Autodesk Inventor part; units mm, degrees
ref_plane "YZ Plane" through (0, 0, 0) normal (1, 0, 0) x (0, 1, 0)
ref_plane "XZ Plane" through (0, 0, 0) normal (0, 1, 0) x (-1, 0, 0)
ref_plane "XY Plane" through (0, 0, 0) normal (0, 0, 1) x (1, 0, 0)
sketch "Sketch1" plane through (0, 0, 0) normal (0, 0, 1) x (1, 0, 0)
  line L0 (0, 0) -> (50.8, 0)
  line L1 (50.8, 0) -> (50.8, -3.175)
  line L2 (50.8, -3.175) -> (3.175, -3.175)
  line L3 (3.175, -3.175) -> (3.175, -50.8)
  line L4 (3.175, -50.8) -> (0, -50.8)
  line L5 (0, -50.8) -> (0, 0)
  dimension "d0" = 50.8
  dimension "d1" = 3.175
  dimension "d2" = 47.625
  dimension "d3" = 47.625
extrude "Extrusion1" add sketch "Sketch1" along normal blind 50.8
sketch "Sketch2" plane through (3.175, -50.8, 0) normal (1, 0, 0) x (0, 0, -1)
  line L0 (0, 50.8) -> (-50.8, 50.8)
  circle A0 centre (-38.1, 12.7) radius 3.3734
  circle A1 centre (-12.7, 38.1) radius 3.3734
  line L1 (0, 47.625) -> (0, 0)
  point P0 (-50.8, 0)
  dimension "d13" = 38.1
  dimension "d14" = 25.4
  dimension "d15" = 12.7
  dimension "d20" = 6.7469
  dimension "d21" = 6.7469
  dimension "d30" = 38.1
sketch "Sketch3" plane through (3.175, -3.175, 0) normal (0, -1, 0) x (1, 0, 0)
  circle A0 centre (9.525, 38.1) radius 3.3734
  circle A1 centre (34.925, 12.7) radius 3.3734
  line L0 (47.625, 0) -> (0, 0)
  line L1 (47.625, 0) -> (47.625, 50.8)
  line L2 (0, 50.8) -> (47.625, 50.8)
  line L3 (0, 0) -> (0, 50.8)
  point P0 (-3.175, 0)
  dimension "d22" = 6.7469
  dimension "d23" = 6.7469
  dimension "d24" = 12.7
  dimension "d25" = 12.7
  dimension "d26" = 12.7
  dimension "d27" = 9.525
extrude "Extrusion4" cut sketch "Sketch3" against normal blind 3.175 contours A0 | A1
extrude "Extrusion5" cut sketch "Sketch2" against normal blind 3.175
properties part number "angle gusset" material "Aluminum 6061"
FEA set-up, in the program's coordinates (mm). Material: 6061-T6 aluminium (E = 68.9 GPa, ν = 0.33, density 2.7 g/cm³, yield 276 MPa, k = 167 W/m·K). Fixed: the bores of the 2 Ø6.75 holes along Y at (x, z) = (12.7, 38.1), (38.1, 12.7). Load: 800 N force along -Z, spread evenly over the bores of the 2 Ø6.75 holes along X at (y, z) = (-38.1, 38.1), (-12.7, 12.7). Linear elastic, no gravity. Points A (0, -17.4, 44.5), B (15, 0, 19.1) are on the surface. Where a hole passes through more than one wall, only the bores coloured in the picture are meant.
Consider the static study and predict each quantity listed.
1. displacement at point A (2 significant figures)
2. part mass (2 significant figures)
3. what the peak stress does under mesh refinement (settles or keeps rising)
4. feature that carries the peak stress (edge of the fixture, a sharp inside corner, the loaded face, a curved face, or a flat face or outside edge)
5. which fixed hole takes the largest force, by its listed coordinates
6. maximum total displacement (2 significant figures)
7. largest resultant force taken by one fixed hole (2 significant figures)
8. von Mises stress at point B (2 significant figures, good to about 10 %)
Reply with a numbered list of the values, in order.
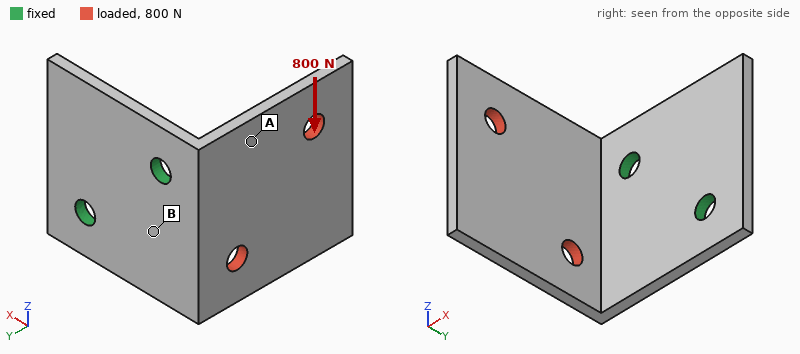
1. 0.19 mm
2. 42 g
3. keeps rising
4. edge of the fixture
5. (12.7, 38.1)
6. 0.80 mm
7. 860 N
8. 63 MPa
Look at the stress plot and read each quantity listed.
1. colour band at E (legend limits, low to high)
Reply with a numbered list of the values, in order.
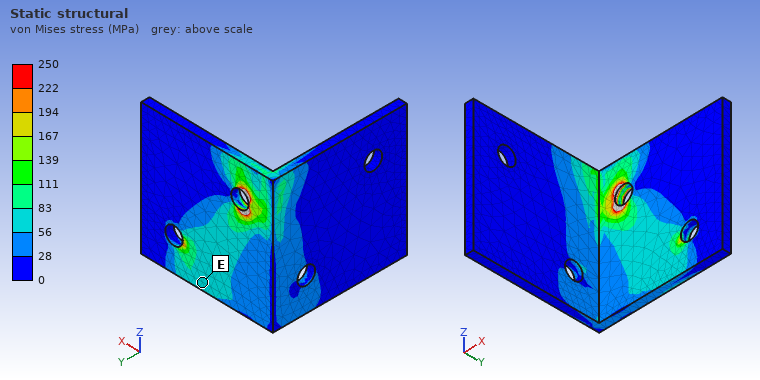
1. 56 to 83 MPa
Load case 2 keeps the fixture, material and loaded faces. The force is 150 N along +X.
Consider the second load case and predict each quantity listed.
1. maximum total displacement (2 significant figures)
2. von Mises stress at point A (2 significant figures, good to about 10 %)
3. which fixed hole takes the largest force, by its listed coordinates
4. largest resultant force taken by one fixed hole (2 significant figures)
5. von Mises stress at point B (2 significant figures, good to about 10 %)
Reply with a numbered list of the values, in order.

1. 0.45 mm
2. 23 MPa
3. (12.7, 38.1)
4. 94 N
5. 18 MPa
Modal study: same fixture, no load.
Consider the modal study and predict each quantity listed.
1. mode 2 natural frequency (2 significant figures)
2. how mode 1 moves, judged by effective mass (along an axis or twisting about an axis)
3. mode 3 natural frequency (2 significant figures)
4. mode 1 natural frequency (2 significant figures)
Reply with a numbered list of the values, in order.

1. 1300 Hz
2. along X
3. 2300 Hz
4. 770 Hz
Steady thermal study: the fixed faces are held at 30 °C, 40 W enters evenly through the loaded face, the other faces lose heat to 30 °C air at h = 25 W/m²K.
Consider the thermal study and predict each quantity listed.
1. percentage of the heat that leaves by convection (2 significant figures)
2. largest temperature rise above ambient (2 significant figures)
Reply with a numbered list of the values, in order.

1. 17 %
2. 62 K
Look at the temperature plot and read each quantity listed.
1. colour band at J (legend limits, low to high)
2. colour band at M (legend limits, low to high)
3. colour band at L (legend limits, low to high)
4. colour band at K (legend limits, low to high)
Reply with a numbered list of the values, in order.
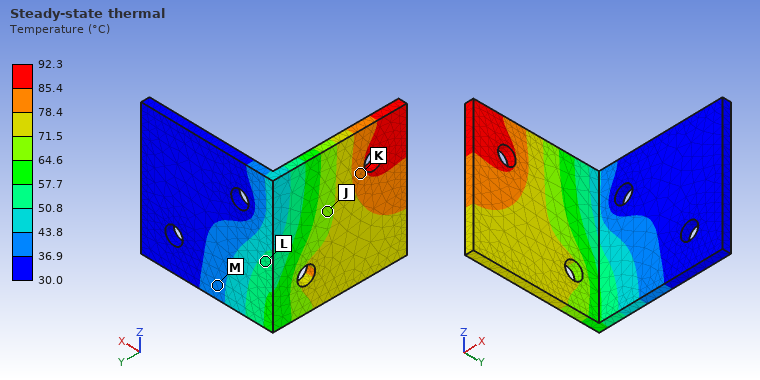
1. 64.6 to 71.5 °C
2. 36.9 to 43.8 °C
3. 50.8 to 57.7 °C
4. 78.4 to 85.4 °C
